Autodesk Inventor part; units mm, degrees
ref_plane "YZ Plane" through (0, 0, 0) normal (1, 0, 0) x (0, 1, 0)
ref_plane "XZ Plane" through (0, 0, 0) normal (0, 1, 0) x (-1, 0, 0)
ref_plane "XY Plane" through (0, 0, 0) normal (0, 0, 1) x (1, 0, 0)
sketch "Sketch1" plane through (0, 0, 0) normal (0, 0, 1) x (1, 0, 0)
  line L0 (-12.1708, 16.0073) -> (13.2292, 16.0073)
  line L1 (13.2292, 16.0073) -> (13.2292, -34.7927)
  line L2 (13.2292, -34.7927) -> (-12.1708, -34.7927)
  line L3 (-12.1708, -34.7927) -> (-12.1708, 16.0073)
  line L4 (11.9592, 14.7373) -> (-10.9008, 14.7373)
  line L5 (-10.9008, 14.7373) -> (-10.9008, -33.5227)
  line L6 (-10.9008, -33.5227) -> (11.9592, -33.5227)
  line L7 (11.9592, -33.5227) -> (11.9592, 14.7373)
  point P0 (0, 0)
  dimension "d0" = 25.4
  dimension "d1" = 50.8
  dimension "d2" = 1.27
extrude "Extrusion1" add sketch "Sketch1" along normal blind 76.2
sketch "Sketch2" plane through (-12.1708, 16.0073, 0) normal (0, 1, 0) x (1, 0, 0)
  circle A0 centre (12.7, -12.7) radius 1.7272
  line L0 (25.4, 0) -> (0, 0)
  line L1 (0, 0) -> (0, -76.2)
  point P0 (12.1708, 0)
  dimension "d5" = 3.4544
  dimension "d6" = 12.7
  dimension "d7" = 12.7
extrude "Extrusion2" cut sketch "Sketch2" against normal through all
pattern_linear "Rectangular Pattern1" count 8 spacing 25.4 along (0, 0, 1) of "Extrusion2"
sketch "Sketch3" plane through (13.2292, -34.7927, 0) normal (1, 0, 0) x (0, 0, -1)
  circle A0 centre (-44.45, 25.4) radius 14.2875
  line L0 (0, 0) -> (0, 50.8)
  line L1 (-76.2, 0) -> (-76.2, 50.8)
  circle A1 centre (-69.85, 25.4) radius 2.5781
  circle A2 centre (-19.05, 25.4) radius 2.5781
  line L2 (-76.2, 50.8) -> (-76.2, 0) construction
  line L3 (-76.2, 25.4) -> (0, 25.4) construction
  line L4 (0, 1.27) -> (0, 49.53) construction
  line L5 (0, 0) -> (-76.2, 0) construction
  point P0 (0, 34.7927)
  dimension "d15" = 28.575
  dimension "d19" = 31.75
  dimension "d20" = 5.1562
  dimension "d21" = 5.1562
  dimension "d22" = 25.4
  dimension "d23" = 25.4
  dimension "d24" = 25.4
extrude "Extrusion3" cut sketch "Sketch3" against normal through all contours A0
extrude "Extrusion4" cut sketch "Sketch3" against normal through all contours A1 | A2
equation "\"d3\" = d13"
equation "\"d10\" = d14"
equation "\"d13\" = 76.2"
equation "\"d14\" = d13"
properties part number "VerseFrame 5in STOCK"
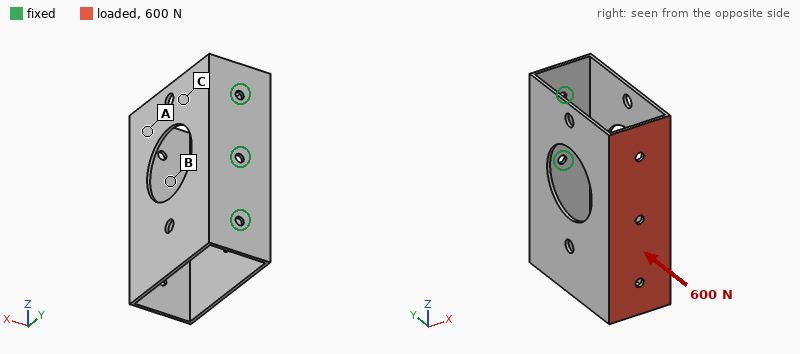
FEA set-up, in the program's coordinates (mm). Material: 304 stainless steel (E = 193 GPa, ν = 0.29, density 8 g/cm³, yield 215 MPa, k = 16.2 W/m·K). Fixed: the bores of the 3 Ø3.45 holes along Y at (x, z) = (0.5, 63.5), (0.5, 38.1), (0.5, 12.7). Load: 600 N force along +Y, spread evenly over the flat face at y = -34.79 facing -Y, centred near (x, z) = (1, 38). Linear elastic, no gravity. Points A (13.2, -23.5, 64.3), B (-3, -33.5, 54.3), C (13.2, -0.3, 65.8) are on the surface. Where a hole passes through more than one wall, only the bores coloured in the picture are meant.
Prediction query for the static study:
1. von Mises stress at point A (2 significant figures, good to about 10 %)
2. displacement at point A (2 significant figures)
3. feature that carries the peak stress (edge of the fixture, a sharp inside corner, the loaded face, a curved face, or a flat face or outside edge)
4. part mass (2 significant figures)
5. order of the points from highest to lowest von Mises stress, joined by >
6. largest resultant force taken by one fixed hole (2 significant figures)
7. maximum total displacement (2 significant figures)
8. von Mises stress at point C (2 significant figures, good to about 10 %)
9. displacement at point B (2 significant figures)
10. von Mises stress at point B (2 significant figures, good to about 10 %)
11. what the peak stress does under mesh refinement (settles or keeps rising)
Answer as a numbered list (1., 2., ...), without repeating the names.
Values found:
1. 12 MPa
2. 63 µm
3. edge of the fixture
4. 100 g
5. B > C > A
6. 210 N
7. 89 µm
8. 23 MPa
9. 81 µm
10. 62 MPa
11. keeps rising
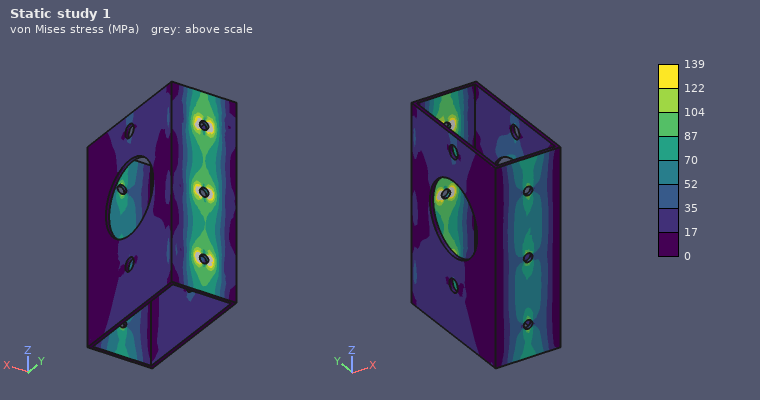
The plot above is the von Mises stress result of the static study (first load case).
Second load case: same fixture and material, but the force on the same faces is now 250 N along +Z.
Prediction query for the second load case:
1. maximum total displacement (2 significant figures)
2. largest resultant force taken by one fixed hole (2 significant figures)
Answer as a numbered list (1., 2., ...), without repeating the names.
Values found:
1. 0.11 mm
2. 240 N
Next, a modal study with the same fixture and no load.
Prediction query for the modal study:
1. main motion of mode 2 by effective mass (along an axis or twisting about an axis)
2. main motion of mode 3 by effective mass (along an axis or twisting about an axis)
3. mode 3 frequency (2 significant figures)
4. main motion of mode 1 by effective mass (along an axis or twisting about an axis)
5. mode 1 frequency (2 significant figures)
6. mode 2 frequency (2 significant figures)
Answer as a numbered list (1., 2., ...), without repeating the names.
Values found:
1. twisting about Y
2. along Z
3. 1100 Hz
4. along X
5. 300 Hz
6. 1000 Hz
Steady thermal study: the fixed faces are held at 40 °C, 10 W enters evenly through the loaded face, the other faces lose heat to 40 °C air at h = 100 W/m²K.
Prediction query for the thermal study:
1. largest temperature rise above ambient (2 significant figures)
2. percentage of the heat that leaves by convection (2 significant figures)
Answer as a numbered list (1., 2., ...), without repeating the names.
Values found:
1. 28 K
2. 100 %
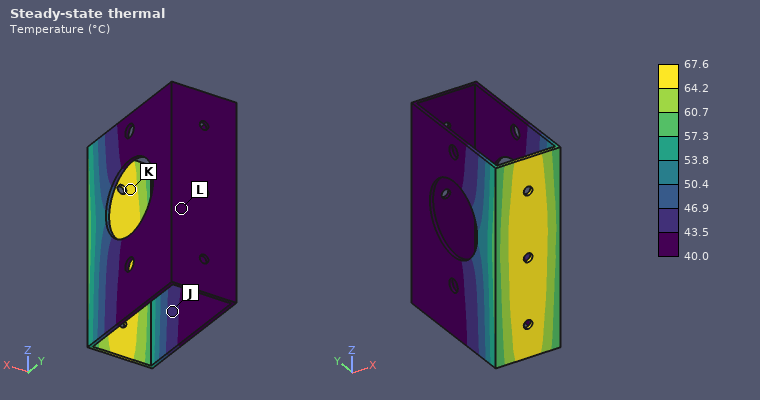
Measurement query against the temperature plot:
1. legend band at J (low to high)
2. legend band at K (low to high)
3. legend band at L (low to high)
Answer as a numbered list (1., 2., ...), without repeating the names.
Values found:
1. 43.5 to 46.9 °C
2. 64.2 to 67.6 °C
3. 40.0 to 43.5 °C
